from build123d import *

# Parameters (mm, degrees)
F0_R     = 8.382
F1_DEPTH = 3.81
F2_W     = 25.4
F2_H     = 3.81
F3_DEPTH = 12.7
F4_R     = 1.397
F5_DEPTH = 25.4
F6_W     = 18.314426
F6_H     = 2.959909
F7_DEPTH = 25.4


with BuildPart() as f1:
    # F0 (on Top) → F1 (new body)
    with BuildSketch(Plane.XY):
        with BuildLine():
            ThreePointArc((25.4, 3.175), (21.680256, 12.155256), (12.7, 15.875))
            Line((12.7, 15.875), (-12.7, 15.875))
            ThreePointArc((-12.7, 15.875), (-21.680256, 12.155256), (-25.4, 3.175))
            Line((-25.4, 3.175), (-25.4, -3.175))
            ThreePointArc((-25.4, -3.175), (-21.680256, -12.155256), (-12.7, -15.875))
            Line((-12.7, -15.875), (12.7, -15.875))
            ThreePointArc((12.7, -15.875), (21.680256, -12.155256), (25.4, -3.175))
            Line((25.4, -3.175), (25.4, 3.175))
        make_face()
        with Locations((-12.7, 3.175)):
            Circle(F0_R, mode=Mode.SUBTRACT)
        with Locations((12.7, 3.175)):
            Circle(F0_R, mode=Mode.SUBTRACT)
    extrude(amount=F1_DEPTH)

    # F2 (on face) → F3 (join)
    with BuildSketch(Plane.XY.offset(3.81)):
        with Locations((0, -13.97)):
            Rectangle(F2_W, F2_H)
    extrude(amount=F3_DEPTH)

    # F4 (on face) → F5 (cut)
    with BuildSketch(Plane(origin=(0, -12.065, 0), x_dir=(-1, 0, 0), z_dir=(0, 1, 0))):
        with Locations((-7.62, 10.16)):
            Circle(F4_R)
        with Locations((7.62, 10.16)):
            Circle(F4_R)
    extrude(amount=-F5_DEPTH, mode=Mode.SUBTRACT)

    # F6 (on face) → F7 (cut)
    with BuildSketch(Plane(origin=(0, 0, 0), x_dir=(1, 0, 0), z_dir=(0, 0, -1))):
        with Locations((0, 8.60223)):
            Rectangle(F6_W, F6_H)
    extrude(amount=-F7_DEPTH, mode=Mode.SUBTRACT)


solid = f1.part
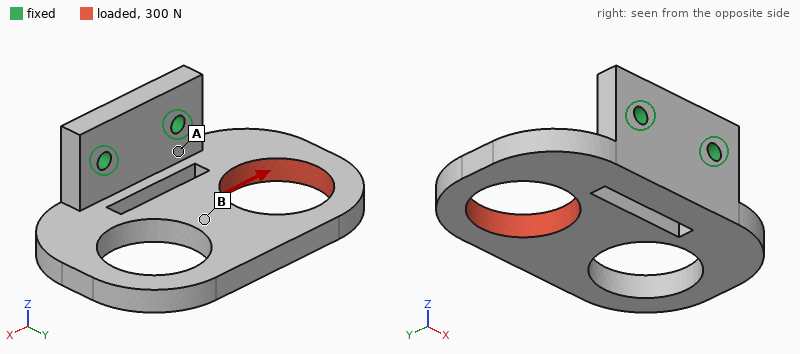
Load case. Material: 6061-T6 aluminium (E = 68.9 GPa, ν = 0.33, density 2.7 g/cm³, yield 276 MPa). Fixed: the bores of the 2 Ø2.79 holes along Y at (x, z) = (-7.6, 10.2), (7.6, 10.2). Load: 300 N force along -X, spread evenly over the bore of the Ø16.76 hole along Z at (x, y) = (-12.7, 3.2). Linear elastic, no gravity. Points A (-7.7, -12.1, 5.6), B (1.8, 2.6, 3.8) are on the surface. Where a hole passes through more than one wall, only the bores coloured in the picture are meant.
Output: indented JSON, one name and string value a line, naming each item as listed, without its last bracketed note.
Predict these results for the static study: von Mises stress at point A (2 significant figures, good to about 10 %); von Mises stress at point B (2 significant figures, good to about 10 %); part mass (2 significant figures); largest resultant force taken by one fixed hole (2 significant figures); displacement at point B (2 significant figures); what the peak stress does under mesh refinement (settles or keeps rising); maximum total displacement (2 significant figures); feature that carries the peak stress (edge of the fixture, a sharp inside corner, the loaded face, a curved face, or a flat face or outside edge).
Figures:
{
  "von Mises stress at point A": "37 MPa",
  "von Mises stress at point B": "12 MPa",
  "part mass": "13 g",
  "largest resultant force taken by one fixed hole": "340 N",
  "displacement at point B": "32 µm",
  "what the peak stress does under mesh refinement": "keeps rising",
  "maximum total displacement": "67 µm",
  "feature that carries the peak stress": "edge of the fixture"
}
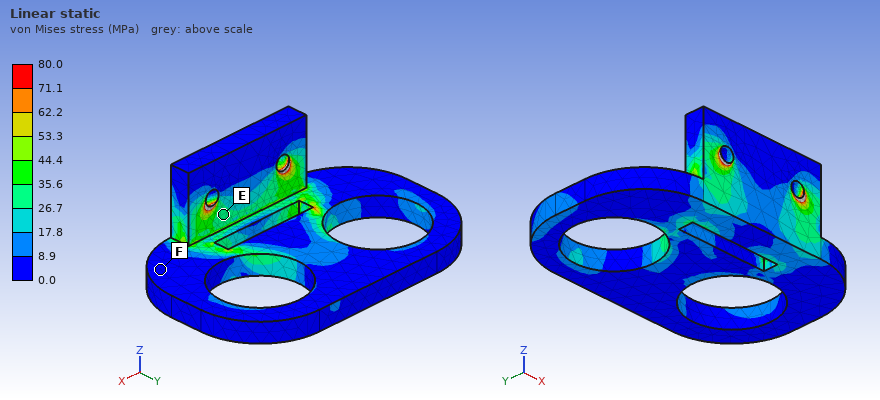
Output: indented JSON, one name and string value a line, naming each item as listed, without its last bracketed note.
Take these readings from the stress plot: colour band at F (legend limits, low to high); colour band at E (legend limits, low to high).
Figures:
{
  "colour band at F": "0.0 to 8.9 MPa",
  "colour band at E": "26.7 to 35.6 MPa"
}
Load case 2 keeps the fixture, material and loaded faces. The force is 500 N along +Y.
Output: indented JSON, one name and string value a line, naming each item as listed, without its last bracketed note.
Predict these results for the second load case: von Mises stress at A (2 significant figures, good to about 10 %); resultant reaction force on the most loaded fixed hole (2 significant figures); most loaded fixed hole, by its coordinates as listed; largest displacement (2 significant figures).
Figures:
{
  "von Mises stress at A": "65 MPa",
  "resultant reaction force on the most loaded fixed hole": "580 N",
  "most loaded fixed hole, by its coordinates as listed": "(-7.6, 10.2)",
  "largest displacement": "0.13 mm"
}
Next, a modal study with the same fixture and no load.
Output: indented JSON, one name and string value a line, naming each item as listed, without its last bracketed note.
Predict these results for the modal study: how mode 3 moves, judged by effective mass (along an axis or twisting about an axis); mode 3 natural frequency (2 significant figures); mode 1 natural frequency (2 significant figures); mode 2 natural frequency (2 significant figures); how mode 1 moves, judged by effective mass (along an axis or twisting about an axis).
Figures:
{
  "how mode 3 moves, judged by effective mass": "along X",
  "mode 3 natural frequency": "4700 Hz",
  "mode 1 natural frequency": "1900 Hz",
  "mode 2 natural frequency": "3600 Hz",
  "how mode 1 moves, judged by effective mass": "along Z"
}
